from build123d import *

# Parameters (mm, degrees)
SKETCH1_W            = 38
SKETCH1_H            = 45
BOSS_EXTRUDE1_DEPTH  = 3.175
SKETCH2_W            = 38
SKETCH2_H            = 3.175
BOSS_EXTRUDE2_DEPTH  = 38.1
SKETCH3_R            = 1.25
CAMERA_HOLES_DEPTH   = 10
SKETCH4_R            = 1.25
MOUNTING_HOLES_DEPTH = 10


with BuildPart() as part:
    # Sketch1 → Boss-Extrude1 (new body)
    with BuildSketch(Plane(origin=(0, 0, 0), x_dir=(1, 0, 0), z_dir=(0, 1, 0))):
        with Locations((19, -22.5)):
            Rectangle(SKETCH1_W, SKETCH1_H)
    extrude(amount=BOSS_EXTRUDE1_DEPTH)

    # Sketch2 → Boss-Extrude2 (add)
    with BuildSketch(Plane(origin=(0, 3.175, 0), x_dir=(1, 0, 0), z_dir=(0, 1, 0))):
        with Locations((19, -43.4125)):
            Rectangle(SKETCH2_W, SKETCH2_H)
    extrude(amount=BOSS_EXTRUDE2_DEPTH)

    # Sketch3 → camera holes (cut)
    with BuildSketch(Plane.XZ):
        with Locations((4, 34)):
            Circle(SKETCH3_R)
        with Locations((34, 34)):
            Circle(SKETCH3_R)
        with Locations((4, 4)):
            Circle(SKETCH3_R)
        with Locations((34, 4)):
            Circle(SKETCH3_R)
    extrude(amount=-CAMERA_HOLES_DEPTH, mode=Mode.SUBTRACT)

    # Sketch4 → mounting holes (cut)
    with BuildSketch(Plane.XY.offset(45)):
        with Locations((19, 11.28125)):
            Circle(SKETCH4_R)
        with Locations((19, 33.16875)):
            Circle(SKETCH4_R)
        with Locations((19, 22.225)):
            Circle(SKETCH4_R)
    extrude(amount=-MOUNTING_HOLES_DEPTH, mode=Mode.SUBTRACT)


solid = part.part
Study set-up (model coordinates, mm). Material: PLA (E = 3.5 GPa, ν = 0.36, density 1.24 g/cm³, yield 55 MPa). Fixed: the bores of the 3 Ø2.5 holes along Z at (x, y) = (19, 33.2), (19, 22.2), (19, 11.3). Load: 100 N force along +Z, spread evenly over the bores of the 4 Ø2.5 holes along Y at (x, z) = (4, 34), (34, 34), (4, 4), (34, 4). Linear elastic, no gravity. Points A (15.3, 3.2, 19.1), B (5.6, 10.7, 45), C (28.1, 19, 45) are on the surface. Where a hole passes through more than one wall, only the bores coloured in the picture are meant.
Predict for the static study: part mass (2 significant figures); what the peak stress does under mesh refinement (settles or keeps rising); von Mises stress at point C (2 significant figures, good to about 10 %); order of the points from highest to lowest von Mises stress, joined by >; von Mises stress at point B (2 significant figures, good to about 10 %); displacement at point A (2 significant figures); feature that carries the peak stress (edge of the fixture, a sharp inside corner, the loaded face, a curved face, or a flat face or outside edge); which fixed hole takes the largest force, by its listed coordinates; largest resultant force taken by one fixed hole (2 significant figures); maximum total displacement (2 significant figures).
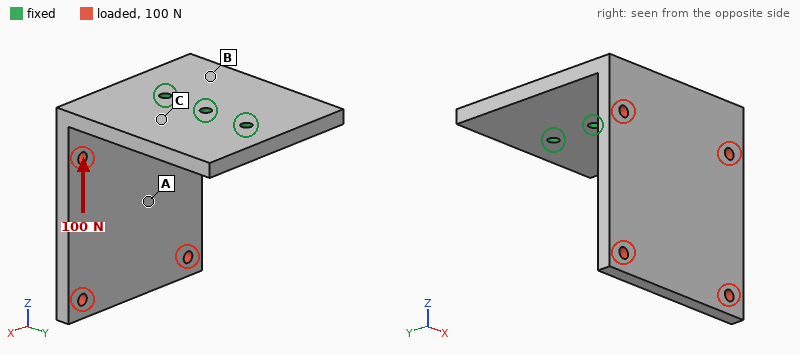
12 g
keeps rising
3.2 MPa
B > C > A
5.7 MPa
0.48 mm
edge of the fixture
(19, 11.3)
140 N
0.85 mm
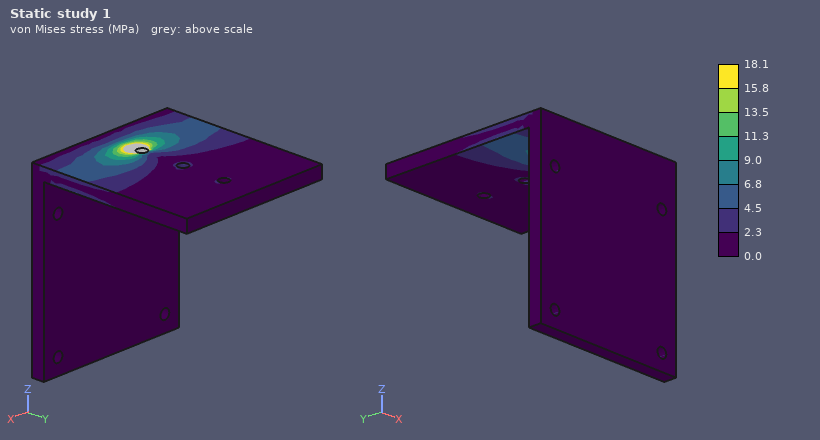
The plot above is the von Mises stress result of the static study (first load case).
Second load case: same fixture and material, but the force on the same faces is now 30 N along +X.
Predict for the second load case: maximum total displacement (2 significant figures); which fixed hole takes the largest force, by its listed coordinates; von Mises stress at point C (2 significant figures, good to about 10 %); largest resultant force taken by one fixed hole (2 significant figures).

0.76 mm
(19, 11.3)
4.3 MPa
40 N
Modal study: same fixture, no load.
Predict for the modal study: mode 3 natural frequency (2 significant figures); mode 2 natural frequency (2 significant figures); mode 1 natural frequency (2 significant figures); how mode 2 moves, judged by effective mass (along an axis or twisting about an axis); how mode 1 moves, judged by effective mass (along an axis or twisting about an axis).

1100 Hz
480 Hz
330 Hz
along X
along Y
